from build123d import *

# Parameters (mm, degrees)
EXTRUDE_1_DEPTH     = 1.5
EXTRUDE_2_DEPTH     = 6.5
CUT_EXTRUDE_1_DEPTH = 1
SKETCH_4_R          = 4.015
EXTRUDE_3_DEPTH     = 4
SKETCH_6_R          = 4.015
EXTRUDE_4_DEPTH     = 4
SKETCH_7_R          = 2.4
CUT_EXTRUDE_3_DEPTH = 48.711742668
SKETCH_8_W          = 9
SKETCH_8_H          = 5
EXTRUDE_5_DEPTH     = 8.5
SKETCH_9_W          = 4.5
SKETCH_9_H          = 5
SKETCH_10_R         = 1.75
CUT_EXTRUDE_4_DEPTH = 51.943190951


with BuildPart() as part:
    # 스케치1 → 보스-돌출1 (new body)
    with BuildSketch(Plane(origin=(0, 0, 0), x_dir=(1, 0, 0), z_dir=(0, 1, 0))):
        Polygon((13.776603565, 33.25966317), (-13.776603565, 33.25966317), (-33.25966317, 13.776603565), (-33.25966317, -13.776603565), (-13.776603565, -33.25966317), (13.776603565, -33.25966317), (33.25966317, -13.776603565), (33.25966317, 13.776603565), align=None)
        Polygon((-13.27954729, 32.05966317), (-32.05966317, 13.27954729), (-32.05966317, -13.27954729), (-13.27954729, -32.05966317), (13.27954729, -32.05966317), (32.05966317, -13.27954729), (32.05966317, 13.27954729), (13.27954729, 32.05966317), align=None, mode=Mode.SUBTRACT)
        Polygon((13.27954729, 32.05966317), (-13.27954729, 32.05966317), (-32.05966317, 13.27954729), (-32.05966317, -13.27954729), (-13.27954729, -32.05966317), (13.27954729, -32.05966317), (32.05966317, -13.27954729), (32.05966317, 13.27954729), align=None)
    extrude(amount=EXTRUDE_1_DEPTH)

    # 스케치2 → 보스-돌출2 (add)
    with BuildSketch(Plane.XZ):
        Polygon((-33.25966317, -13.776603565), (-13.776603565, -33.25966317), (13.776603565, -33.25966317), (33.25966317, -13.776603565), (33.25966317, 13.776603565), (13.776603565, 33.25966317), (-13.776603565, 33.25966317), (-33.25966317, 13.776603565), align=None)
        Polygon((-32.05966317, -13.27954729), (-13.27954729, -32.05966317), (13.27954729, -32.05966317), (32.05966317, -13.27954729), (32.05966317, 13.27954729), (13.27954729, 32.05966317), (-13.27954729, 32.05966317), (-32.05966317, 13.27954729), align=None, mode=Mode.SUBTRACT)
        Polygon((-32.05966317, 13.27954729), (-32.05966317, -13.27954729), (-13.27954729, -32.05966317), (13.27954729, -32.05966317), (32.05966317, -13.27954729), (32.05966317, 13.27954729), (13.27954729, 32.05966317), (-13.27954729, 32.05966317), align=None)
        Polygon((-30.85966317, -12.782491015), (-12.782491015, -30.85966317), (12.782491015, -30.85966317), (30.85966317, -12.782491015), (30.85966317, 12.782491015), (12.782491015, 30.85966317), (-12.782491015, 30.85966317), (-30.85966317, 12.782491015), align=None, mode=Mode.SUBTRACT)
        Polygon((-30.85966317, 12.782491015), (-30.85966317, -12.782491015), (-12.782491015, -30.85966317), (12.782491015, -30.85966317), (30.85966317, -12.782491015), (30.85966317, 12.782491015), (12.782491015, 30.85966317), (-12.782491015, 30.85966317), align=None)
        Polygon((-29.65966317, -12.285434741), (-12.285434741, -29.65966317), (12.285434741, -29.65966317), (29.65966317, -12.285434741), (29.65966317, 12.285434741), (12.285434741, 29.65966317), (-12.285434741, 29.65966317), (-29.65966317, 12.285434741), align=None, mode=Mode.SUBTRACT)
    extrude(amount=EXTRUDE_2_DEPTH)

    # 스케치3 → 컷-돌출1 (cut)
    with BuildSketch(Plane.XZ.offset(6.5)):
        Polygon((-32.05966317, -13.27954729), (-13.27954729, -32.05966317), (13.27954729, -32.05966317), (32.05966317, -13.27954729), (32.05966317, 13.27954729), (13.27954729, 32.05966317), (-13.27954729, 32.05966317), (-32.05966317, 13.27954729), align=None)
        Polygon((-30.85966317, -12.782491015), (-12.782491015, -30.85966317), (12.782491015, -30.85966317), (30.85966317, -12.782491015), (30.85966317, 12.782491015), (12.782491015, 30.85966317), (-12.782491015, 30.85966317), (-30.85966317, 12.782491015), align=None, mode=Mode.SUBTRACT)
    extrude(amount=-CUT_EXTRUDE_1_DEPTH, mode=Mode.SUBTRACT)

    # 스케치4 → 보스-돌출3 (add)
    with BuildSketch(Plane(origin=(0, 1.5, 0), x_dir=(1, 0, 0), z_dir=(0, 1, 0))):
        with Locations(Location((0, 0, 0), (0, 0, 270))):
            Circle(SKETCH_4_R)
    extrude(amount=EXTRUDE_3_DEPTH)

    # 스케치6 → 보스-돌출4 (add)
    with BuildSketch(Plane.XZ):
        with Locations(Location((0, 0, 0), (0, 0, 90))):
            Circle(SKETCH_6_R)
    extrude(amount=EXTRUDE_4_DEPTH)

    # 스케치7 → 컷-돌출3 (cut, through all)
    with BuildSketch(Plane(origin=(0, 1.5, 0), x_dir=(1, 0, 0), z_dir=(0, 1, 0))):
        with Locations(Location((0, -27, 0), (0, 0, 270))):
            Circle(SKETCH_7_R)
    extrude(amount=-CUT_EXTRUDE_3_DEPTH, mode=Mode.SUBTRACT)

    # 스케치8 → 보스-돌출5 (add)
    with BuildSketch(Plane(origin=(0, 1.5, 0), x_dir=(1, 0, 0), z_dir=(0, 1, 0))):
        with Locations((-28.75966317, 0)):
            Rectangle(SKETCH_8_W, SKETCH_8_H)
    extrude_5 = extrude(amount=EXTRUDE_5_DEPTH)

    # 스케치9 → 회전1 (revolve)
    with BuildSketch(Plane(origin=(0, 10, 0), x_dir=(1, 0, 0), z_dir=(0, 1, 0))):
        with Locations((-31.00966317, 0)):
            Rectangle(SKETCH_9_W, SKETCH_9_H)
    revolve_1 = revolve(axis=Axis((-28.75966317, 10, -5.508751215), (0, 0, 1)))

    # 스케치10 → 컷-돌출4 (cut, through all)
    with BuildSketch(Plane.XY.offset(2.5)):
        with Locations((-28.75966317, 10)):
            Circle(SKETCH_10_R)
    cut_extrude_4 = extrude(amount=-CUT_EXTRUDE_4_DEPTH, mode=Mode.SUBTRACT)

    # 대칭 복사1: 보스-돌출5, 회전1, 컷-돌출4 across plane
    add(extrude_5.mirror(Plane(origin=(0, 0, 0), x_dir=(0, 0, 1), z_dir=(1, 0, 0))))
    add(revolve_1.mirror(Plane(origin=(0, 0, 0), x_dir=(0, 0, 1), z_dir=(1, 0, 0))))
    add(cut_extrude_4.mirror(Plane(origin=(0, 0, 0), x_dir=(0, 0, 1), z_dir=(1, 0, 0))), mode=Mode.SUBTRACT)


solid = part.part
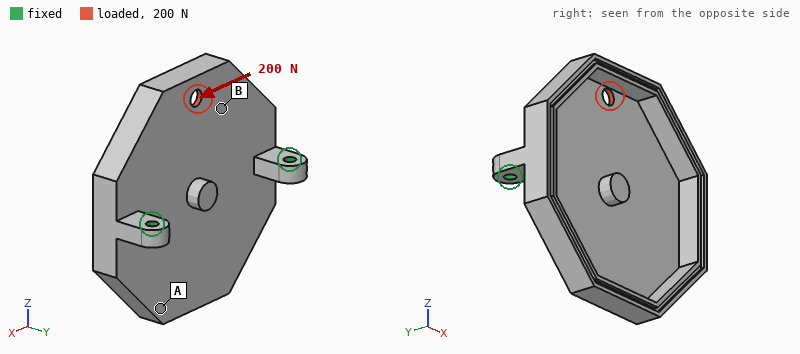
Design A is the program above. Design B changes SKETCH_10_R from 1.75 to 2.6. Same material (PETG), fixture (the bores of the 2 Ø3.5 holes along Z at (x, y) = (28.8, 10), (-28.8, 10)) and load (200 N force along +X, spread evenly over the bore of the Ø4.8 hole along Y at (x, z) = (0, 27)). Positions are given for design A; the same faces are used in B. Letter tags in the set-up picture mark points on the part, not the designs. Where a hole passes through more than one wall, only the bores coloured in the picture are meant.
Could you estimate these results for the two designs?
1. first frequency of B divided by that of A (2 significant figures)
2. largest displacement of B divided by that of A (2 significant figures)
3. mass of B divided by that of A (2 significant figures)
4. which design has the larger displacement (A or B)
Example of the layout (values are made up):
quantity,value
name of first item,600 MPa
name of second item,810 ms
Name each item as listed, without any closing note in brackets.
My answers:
quantity,value
first frequency of B divided by that of A,1.0
largest displacement of B divided by that of A,0.79
mass of B divided by that of A,0.99
which design has the larger displacement,A
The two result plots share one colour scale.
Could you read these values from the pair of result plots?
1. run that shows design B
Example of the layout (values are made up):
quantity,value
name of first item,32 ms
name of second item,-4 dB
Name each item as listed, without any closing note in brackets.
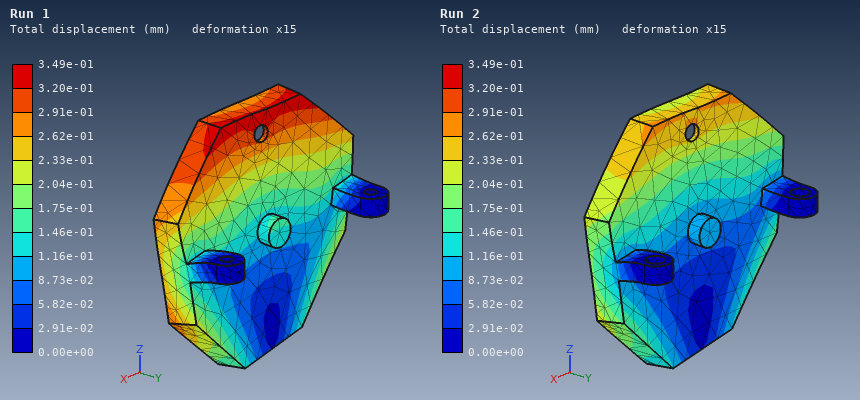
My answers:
quantity,value
run that shows design B,Run 2
